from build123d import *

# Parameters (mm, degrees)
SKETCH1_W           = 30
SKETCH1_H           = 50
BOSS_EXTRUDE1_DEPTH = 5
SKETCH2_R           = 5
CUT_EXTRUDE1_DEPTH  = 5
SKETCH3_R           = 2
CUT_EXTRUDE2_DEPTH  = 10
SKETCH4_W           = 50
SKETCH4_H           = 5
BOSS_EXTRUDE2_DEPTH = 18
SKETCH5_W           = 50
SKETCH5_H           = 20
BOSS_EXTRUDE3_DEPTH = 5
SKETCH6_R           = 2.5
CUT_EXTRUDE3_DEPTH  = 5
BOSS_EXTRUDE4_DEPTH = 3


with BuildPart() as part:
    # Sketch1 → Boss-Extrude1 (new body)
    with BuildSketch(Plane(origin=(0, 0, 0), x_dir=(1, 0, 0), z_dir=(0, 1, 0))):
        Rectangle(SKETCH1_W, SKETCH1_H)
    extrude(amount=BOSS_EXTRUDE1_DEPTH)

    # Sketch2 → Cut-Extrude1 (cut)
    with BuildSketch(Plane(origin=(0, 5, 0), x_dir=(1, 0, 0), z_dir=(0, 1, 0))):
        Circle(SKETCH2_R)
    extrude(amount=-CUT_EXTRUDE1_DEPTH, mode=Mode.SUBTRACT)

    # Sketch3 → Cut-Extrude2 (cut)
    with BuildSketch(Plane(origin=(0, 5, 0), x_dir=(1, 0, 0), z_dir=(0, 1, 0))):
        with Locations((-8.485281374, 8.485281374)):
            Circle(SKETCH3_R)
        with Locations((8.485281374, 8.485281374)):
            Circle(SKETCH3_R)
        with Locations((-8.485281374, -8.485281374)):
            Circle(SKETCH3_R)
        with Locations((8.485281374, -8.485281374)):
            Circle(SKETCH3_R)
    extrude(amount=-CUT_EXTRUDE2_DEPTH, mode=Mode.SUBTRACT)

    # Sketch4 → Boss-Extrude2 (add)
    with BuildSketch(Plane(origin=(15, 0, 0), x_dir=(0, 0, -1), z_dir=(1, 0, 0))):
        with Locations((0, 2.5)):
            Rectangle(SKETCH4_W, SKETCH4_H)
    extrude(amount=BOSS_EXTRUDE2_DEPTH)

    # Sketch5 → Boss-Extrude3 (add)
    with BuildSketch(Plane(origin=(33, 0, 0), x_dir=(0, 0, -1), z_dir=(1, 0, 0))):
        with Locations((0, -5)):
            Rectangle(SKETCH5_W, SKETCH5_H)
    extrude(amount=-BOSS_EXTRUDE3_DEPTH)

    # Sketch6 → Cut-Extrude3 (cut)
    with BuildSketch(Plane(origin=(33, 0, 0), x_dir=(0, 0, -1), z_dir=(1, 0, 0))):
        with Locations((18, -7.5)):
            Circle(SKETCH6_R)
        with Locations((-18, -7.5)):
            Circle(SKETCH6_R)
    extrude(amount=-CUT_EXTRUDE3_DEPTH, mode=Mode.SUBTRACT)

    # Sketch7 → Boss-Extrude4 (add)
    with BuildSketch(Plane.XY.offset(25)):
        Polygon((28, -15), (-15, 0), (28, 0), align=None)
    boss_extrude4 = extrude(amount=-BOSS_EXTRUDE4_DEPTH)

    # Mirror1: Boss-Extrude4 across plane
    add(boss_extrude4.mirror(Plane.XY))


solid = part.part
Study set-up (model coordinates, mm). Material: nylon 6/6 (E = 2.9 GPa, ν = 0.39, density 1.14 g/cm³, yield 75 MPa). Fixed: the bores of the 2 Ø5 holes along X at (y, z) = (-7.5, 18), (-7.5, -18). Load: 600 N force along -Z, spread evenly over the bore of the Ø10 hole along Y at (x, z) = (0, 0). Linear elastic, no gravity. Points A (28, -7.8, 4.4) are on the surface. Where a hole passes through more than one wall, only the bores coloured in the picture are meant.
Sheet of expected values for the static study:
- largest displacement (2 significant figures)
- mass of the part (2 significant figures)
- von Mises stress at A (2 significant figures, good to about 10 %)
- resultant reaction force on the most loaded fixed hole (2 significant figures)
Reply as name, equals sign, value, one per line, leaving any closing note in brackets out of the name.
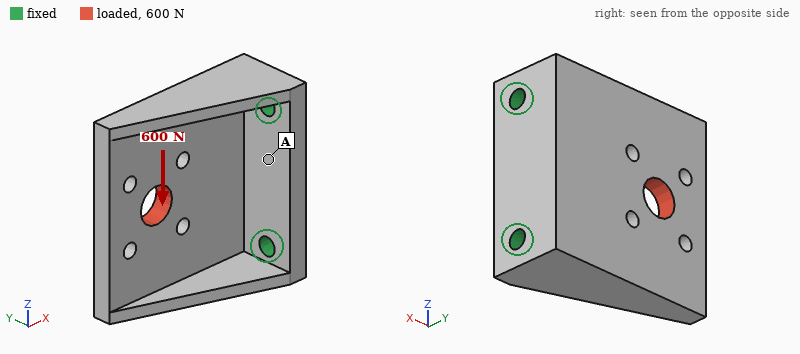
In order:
largest displacement = 0.80 mm
mass of the part = 19 g
von Mises stress at A = 5.8 MPa
resultant reaction force on the most loaded fixed hole = 560 N
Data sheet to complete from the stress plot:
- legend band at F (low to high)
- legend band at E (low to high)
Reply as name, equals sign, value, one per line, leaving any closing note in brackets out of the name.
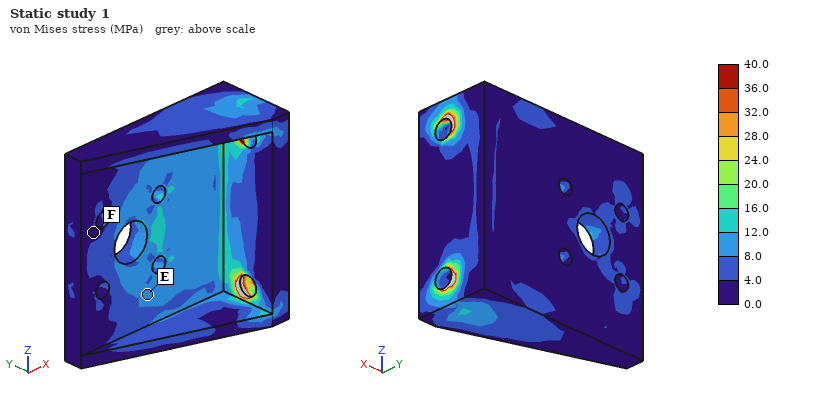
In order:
legend band at F = 0.0 to 4.0 MPa
legend band at E = 8.0 to 12.0 MPa
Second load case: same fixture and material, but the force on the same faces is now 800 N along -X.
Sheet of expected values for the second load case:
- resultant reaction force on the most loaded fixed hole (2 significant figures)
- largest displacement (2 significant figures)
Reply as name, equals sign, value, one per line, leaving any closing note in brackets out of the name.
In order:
resultant reaction force on the most loaded fixed hole = 400 N
largest displacement = 0.86 mm
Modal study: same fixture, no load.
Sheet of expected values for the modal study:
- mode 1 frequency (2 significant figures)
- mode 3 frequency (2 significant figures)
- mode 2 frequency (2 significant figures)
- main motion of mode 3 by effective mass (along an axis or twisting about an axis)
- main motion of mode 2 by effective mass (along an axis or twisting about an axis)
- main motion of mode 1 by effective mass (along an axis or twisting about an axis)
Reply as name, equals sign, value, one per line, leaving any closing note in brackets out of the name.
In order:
mode 1 frequency = 860 Hz
mode 3 frequency = 2900 Hz
mode 2 frequency = 1400 Hz
main motion of mode 3 by effective mass = along Z
main motion of mode 2 by effective mass = along Z
main motion of mode 1 by effective mass = along Y
